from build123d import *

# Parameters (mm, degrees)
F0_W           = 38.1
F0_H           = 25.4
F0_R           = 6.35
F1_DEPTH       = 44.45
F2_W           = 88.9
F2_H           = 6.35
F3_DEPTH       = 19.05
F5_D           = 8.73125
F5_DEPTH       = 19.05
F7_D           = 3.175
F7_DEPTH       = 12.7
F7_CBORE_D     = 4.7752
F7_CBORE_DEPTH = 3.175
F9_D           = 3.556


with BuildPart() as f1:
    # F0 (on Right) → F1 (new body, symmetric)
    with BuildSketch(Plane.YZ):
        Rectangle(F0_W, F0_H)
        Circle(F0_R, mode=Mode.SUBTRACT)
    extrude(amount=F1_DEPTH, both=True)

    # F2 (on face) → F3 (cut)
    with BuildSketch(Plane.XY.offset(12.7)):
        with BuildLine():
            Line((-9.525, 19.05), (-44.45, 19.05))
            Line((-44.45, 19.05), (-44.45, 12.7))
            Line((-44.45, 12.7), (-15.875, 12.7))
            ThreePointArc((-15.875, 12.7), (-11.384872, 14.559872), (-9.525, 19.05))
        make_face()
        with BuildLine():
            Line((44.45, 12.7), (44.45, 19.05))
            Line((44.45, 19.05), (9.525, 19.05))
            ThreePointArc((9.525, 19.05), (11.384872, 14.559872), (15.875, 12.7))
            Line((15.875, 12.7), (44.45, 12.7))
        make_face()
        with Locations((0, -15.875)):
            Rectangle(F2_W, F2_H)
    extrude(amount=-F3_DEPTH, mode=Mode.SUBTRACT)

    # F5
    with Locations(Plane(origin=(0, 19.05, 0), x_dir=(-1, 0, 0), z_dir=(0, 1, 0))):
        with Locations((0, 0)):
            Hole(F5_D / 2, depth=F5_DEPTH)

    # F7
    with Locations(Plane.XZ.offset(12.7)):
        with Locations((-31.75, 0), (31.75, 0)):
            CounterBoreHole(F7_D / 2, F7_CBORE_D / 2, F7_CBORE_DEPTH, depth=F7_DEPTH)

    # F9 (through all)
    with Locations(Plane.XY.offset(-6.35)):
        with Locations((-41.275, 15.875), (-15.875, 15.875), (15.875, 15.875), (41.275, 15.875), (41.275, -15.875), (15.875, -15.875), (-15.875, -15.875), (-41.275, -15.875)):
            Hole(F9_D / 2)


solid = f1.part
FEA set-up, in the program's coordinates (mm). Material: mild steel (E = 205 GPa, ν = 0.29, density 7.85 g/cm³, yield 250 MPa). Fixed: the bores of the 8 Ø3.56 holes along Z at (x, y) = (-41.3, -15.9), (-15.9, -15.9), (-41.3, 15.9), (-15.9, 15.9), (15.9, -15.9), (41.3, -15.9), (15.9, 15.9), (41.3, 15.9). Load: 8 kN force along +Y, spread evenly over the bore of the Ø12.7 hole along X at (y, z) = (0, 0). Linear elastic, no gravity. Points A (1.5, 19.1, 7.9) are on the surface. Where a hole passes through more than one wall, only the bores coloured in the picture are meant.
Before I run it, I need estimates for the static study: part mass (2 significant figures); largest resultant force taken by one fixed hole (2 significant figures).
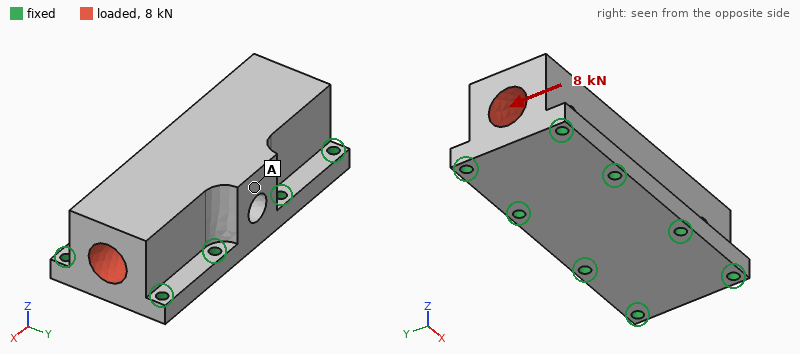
430 g
1.5 kN
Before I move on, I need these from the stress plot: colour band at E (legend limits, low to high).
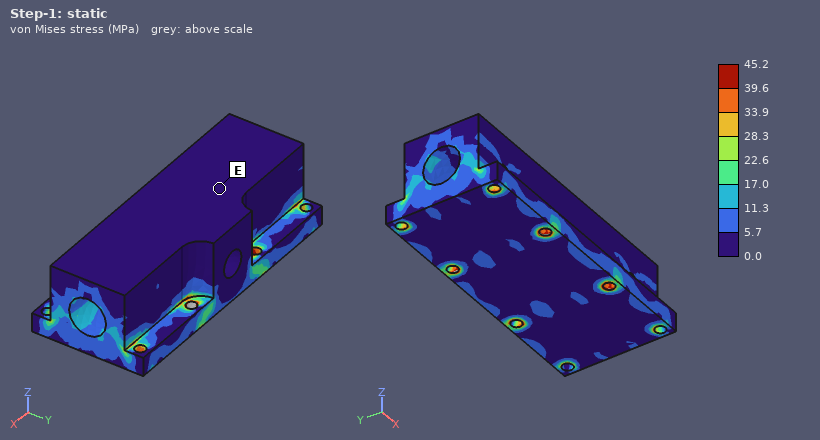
0.0 to 5.7 MPa
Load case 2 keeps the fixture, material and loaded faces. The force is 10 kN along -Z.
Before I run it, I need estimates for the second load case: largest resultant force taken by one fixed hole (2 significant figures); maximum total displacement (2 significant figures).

1.6 kN
2.8 µm
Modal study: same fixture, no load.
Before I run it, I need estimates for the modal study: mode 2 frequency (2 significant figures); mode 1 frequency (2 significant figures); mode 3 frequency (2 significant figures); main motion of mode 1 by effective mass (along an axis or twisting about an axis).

17 kHz
14 kHz
18 kHz
along Y
